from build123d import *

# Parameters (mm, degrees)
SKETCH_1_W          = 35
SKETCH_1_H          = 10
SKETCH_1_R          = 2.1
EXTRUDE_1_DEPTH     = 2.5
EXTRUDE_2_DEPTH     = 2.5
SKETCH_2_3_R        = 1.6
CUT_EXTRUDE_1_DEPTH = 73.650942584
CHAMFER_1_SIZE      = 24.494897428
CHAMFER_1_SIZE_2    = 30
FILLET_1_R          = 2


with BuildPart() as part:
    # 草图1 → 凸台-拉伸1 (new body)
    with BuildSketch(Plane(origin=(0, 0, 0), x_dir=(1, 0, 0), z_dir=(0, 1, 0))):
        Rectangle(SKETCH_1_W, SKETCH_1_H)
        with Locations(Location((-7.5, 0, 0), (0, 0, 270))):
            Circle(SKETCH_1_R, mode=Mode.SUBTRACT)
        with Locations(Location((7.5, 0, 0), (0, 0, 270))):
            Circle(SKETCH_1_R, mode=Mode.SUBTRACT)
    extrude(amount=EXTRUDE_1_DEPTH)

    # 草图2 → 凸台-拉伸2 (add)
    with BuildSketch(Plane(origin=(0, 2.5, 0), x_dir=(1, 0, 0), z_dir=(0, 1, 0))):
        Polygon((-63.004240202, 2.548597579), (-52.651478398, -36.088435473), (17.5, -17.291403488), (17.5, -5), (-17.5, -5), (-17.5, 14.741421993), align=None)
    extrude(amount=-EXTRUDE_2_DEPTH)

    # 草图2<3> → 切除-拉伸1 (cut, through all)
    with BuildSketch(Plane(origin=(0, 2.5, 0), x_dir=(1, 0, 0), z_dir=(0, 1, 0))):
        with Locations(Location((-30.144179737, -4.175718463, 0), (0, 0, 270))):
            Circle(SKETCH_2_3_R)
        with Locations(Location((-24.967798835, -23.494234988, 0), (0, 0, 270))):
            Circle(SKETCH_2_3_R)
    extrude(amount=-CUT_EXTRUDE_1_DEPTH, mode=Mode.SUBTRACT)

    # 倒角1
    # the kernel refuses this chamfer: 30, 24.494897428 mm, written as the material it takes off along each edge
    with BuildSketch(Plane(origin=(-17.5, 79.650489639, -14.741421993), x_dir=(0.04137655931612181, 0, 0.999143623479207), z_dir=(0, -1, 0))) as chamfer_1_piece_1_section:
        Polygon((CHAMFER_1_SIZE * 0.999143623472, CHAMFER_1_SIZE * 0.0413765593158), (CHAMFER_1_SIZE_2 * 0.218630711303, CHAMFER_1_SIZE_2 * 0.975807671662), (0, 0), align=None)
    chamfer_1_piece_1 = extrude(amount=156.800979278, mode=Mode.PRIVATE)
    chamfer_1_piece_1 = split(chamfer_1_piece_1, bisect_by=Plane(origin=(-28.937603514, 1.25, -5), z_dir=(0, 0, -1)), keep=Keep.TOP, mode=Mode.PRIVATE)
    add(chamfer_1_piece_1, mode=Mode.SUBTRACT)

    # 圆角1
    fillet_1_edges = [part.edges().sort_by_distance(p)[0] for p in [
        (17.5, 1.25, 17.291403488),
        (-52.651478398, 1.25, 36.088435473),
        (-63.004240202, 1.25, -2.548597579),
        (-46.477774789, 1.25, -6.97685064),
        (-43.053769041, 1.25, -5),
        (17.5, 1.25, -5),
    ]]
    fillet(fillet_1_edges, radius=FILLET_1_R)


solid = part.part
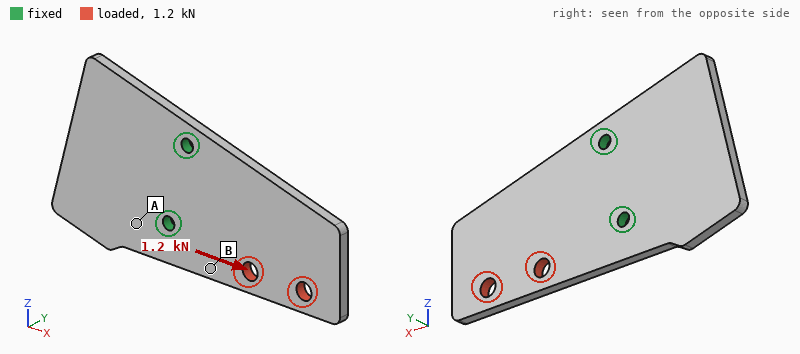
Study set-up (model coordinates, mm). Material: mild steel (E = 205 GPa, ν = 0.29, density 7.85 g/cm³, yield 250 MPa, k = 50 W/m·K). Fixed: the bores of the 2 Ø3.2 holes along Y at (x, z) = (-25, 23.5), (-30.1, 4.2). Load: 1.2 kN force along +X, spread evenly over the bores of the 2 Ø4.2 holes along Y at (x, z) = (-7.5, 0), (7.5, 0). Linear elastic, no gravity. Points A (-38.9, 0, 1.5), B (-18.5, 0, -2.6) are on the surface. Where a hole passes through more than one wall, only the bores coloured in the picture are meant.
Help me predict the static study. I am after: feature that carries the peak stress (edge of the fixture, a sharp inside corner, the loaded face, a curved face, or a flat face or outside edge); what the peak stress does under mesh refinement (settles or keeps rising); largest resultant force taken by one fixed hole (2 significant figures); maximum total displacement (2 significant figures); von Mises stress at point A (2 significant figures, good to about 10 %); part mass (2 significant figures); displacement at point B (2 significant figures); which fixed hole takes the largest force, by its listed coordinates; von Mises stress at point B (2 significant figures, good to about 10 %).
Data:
edge of the fixture
keeps rising
1.4 kN
15 µm
8.0 MPa
47 g
3.7 µm
(-30.1, 4.2)
39 MPa
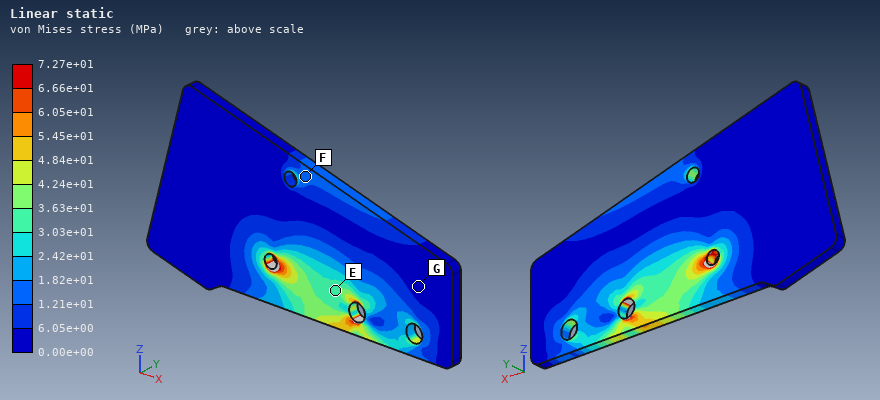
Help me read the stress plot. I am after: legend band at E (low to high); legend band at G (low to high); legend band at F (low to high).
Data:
3.03e+01 to 3.63e+01 MPa
0.00e+00 to 6.05e+00 MPa
1.21e+01 to 1.82e+01 MPa
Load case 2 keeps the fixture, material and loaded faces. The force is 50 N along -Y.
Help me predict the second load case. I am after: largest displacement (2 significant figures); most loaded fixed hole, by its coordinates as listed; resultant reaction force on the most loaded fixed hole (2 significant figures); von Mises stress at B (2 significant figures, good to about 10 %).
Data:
0.11 mm
(-30.1, 4.2)
38 N
28 MPa
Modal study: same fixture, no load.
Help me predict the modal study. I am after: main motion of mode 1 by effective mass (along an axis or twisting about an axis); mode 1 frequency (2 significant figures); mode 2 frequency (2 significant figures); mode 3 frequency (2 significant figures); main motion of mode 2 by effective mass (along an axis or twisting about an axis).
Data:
along Y
1100 Hz
2200 Hz
4100 Hz
along Y
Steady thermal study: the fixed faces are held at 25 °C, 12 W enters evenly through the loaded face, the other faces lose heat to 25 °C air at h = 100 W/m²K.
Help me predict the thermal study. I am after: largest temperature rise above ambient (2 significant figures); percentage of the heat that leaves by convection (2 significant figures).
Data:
59 K
64 %
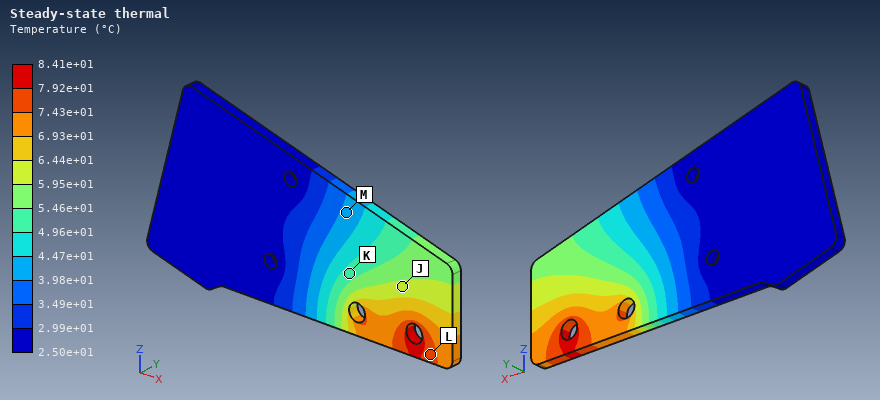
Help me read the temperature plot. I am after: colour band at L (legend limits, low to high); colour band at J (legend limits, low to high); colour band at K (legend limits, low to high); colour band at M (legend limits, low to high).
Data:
7.43e+01 to 7.92e+01 °C
5.95e+01 to 6.44e+01 °C
4.96e+01 to 5.46e+01 °C
3.98e+01 to 4.47e+01 °C
